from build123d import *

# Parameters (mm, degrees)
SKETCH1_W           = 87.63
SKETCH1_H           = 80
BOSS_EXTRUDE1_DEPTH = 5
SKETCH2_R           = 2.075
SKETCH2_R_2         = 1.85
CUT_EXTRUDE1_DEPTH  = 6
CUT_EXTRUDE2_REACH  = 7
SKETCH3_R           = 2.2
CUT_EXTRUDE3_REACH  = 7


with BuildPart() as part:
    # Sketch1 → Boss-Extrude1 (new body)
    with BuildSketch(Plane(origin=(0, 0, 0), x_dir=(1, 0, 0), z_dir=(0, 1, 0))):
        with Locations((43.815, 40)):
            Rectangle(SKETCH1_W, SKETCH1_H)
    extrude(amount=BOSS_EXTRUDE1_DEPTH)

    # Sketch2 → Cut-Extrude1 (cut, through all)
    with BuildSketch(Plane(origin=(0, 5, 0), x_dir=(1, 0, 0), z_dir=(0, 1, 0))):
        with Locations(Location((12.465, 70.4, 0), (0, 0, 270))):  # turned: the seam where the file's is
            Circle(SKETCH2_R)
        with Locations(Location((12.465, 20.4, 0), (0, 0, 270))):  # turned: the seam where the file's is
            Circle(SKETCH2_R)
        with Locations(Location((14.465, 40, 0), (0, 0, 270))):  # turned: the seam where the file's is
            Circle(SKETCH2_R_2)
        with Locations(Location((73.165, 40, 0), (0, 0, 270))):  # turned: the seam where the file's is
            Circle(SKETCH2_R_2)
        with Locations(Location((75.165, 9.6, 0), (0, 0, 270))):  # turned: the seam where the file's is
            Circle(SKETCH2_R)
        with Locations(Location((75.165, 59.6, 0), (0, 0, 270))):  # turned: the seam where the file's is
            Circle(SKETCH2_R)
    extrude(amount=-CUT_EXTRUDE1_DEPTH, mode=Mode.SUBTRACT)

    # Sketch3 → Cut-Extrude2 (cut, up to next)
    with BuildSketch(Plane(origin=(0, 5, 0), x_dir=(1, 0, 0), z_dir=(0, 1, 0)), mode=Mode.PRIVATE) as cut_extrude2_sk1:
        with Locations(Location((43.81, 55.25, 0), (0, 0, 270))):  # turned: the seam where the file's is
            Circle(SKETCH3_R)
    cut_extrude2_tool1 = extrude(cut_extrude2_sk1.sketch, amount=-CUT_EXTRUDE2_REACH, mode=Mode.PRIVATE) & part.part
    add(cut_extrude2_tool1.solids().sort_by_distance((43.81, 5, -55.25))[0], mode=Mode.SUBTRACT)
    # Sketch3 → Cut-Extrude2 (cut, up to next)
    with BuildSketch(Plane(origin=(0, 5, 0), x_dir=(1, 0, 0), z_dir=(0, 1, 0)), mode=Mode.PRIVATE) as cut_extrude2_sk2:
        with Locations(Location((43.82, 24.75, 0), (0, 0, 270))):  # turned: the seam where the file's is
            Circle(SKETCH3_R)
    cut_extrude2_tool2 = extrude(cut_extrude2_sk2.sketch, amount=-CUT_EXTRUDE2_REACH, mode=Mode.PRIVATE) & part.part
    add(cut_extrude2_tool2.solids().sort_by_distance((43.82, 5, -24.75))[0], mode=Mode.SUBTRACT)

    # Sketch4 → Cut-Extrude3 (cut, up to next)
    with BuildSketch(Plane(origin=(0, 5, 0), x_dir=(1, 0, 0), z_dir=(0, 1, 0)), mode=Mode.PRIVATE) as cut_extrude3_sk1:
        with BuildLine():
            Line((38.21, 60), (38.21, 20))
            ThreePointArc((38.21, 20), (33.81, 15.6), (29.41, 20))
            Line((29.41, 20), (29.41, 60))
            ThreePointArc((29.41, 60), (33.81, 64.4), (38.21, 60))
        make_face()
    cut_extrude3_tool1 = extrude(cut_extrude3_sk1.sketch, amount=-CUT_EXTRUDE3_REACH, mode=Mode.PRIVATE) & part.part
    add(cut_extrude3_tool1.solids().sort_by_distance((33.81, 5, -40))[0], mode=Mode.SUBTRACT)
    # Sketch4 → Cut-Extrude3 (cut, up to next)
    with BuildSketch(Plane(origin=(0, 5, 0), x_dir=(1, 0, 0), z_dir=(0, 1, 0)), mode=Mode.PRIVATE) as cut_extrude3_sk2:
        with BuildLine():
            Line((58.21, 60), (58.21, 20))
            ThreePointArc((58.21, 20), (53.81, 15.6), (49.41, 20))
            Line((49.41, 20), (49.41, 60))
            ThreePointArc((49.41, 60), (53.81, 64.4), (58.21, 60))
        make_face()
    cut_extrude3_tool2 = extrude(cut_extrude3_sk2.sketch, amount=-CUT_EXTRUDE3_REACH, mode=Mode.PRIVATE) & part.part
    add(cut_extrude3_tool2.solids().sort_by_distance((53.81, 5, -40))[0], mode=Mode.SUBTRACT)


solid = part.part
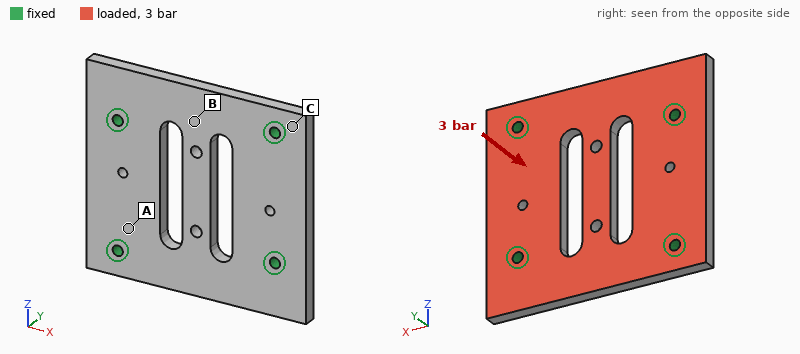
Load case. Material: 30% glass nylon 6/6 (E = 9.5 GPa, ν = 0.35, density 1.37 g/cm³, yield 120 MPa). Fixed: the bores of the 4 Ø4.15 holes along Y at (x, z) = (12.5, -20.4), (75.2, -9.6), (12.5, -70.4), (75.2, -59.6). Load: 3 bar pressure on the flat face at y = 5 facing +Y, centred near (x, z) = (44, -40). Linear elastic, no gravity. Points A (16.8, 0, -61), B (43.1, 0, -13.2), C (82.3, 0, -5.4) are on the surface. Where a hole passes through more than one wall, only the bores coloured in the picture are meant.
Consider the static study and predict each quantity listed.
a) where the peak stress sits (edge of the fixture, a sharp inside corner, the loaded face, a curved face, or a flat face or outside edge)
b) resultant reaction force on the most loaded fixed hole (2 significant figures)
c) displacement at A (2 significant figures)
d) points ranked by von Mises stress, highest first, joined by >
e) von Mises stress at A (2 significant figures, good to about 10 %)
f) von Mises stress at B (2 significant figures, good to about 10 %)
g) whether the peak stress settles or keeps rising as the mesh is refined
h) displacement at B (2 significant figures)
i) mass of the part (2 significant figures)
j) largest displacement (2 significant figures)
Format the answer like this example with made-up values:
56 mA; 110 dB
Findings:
edge of the fixture; 510 N; 0.048 mm; B > A > C; 9.9 MPa; 18 MPa; keeps rising; 0.20 mm; 42 g; 0.32 mm
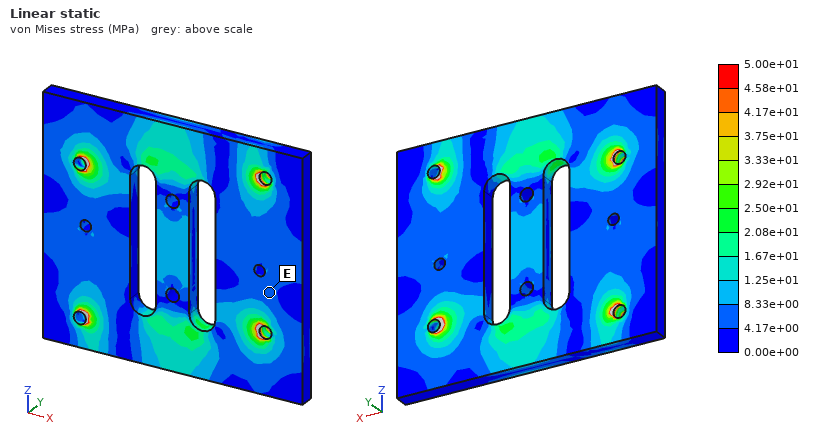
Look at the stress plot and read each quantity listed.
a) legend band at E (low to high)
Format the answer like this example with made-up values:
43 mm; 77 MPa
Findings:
4.17e+00 to 8.33e+00 MPa
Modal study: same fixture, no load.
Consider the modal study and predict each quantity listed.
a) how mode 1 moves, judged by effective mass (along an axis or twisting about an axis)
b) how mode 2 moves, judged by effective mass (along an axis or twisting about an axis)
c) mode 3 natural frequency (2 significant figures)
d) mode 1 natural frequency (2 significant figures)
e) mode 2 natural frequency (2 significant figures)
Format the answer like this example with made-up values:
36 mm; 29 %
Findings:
along Y; twisting about X; 3400 Hz; 2300 Hz; 3000 Hz
